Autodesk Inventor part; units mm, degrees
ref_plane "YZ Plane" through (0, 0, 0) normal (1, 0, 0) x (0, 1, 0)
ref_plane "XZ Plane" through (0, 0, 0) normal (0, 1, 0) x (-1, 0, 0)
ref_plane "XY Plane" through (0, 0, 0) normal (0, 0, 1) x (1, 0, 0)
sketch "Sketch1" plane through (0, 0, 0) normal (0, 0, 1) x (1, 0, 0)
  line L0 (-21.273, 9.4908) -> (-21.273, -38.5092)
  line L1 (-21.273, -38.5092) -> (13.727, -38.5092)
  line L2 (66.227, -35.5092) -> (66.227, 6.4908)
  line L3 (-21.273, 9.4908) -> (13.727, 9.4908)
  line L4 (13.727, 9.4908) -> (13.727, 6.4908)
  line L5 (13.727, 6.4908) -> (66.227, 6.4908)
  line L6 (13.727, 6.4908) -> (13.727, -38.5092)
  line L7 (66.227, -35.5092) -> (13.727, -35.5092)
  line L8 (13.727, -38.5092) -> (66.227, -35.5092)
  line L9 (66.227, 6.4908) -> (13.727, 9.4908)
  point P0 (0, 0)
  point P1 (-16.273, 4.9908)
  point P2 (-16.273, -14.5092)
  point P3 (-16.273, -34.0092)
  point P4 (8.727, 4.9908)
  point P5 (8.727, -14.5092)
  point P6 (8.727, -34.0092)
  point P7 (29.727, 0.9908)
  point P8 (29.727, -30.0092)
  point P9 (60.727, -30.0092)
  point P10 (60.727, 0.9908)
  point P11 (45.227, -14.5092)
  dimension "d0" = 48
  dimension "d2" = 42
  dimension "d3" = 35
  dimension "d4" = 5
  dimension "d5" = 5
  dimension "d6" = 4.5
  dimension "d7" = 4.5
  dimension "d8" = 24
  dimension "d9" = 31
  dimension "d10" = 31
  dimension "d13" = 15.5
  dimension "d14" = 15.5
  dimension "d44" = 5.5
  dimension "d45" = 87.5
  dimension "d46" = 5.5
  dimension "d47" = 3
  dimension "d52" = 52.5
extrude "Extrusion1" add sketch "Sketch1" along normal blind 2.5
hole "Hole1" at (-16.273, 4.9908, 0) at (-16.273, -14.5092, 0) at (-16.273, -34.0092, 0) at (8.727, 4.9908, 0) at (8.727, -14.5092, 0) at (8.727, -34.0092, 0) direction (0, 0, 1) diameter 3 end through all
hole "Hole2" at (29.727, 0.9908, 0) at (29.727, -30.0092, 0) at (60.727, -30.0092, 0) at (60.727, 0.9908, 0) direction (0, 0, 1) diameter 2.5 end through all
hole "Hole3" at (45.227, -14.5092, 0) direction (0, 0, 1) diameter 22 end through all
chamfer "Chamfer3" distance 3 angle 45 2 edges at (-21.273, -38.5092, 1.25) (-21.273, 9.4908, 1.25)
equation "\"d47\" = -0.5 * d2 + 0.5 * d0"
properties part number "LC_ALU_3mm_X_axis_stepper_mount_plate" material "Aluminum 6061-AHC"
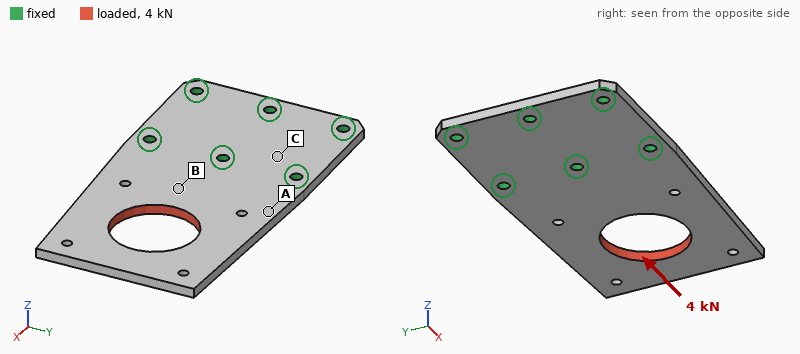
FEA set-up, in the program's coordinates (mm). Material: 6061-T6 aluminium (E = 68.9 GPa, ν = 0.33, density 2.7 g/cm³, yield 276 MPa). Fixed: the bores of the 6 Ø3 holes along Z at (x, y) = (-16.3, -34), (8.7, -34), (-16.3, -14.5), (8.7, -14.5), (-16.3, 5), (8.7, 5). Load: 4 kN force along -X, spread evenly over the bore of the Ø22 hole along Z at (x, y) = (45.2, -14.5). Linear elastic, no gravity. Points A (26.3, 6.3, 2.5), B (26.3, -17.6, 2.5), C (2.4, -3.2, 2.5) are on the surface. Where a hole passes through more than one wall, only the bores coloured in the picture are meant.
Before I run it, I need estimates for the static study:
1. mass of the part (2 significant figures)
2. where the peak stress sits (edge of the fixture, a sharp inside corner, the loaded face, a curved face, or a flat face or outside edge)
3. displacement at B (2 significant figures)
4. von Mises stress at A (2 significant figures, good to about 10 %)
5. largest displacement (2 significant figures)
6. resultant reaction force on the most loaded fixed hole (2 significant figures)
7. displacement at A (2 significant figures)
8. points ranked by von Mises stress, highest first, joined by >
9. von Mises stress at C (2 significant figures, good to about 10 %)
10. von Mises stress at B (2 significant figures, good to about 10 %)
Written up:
24 g
a curved face
8.3 µm
47 MPa
46 µm
1.2 kN
13 µm
A > B > C
11 MPa
27 MPa
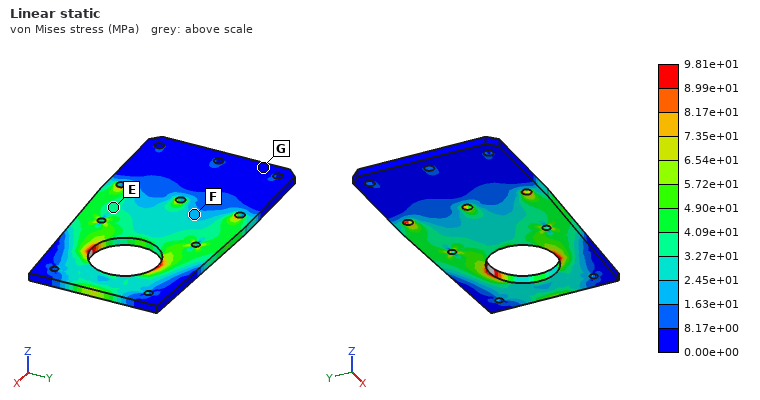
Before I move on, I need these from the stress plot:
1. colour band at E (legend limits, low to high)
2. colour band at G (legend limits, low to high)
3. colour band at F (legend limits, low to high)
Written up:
3.27e+01 to 4.09e+01 MPa
0.00e+00 to 8.17e+00 MPa
1.63e+01 to 2.45e+01 MPa
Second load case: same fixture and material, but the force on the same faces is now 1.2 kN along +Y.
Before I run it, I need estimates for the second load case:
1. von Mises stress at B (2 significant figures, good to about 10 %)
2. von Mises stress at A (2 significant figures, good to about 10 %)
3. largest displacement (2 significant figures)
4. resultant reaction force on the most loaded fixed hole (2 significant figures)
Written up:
35 MPa
33 MPa
68 µm
1.1 kN
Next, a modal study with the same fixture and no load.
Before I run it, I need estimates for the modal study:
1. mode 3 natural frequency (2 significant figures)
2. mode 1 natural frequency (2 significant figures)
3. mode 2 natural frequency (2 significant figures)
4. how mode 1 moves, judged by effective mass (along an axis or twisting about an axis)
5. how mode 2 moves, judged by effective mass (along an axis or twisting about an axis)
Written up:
3600 Hz
690 Hz
1800 Hz
along Z
twisting about X
